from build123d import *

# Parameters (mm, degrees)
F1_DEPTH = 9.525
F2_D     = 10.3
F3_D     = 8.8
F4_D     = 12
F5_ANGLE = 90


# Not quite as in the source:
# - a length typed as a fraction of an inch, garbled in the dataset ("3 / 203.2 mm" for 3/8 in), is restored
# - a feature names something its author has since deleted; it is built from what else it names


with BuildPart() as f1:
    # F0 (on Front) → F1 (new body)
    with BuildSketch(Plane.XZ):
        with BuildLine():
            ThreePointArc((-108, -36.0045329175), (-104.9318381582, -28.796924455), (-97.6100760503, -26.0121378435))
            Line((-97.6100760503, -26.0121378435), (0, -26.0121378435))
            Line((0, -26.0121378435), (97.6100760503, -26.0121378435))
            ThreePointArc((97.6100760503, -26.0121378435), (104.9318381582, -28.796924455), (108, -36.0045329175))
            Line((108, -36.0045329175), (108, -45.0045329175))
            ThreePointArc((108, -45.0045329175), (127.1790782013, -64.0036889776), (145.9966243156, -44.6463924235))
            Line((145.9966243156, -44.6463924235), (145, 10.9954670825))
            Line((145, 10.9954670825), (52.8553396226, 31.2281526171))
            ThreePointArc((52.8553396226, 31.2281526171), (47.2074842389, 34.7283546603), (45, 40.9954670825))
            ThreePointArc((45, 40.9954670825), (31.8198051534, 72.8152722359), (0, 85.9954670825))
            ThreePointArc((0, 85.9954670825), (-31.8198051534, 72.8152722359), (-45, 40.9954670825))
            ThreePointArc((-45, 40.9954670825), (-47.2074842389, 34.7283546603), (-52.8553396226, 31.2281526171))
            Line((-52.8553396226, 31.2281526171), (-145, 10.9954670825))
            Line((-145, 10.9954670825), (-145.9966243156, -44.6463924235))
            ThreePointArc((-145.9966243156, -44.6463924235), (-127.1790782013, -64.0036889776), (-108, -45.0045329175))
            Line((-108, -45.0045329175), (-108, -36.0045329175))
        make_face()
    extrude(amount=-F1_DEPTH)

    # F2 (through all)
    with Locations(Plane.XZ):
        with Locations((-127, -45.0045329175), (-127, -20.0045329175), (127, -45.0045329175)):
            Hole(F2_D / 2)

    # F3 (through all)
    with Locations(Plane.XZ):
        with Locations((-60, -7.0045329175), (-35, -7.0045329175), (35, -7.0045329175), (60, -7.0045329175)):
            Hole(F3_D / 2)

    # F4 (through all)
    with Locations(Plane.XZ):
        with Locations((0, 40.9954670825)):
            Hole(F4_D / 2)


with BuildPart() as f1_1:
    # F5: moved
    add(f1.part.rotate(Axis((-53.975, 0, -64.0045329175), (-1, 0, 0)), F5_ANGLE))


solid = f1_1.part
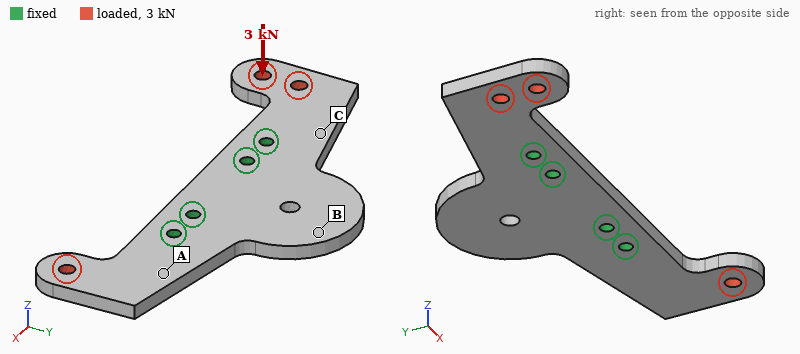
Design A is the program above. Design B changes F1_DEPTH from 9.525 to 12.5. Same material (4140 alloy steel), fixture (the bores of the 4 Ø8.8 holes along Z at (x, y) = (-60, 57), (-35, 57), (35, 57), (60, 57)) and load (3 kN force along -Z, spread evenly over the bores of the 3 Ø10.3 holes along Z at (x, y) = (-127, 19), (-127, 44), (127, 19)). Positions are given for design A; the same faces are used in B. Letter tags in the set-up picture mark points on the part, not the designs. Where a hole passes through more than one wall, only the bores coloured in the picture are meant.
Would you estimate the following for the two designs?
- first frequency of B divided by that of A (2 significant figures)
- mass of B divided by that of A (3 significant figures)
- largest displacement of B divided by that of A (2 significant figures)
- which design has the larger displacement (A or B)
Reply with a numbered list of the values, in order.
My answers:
1. 1.3
2. 1.31
3. 0.46
4. A
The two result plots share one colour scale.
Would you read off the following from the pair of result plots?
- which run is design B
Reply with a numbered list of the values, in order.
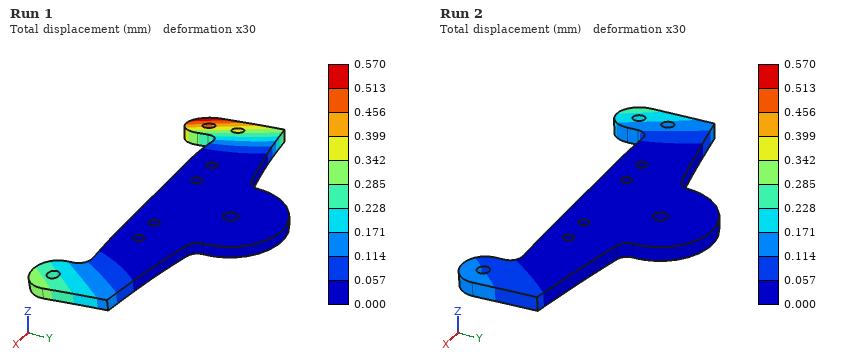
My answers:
1. Run 2
